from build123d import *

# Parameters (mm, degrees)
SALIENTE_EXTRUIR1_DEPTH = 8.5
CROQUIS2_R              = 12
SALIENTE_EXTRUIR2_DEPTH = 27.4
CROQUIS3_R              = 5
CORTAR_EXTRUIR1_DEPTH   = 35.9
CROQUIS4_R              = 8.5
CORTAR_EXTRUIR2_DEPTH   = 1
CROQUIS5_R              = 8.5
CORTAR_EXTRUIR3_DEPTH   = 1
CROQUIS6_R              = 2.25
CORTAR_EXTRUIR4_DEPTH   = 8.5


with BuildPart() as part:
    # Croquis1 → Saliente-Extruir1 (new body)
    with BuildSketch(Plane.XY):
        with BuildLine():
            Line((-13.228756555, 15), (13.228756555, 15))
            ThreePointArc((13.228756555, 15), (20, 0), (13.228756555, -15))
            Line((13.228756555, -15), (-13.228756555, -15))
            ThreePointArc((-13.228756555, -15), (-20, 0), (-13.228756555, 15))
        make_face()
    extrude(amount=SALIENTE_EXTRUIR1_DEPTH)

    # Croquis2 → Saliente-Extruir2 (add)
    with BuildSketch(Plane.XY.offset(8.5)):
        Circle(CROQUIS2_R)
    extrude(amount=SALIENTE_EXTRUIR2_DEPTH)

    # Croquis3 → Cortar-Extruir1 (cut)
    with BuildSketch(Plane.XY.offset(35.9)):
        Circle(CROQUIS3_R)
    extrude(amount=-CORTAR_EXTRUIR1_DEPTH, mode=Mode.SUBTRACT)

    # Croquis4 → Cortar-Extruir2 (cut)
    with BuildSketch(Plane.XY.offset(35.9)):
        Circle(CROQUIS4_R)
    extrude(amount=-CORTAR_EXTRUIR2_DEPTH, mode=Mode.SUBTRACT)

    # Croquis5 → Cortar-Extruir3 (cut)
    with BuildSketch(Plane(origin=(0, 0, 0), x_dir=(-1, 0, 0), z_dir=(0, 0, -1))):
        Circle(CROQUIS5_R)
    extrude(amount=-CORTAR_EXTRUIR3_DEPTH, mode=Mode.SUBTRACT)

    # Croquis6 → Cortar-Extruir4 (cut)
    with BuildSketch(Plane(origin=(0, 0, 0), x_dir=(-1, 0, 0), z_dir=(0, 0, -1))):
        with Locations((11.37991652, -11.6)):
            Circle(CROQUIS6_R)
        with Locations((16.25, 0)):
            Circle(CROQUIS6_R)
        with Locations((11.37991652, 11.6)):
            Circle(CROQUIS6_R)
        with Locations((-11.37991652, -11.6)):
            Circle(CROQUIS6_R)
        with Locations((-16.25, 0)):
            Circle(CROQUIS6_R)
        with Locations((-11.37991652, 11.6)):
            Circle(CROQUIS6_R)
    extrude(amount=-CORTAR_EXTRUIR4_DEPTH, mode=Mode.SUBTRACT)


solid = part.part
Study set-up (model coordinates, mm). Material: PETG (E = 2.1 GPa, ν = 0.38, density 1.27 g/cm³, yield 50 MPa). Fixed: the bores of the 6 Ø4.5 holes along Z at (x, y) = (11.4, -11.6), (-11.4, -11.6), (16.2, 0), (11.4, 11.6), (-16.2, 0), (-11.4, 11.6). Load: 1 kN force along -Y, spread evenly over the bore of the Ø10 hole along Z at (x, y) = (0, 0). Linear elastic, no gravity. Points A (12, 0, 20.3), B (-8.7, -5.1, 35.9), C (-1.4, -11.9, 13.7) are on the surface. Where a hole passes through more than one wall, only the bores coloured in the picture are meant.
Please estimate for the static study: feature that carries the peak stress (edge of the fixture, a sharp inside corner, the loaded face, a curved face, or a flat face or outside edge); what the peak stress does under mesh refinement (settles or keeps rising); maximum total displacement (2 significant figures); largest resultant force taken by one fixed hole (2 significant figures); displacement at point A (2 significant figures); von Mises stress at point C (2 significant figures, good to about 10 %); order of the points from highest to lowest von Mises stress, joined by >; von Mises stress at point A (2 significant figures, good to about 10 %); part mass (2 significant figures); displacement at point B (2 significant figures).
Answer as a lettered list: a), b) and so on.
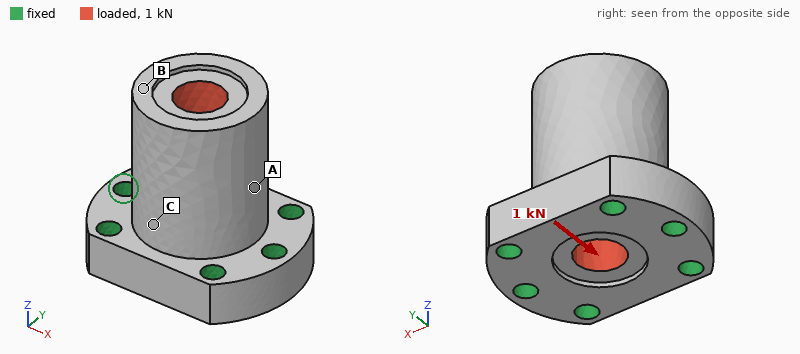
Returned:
a) edge of the fixture
b) keeps rising
c) 0.22 mm
d) 390 N
e) 0.097 mm
f) 4.7 MPa
g) C > A > B
h) 2.7 MPa
i) 22 g
j) 0.20 mm
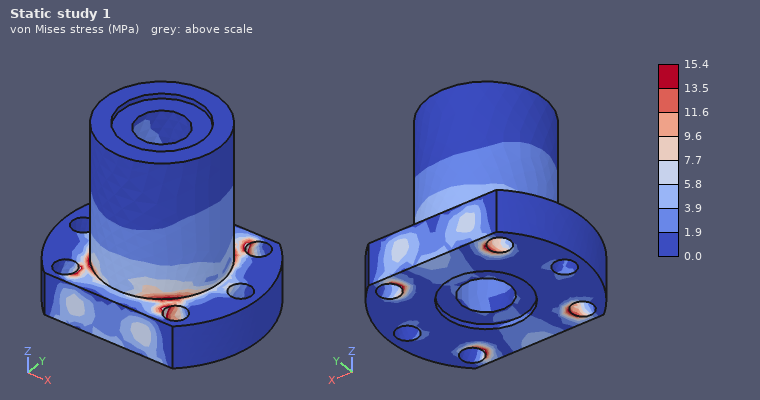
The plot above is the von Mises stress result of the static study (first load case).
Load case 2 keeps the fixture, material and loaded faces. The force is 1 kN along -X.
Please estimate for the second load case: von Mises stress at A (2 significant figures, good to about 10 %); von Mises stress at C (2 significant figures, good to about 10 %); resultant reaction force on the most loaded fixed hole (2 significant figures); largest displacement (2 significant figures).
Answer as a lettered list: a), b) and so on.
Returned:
a) 2.2 MPa
b) 3.2 MPa
c) 330 N
d) 0.17 mm
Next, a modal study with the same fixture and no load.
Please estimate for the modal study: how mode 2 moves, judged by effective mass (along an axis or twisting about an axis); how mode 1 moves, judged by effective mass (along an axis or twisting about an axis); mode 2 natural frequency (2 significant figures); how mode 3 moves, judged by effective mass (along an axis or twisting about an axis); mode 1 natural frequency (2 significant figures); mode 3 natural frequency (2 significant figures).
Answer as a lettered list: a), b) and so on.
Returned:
a) along X
b) along Y
c) 3500 Hz
d) twisting about Z
e) 3100 Hz
f) 6400 Hz
